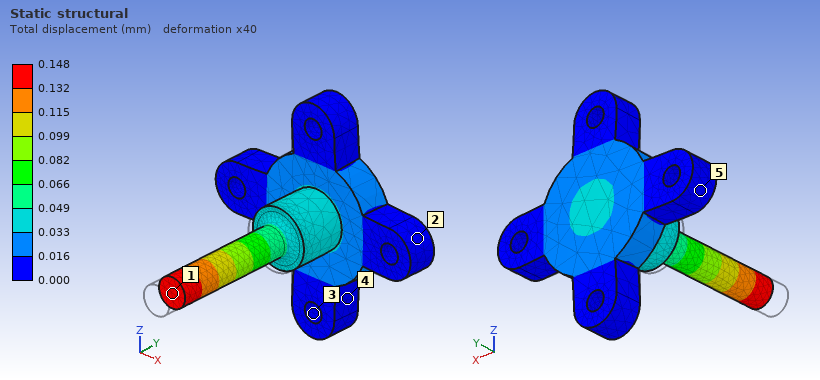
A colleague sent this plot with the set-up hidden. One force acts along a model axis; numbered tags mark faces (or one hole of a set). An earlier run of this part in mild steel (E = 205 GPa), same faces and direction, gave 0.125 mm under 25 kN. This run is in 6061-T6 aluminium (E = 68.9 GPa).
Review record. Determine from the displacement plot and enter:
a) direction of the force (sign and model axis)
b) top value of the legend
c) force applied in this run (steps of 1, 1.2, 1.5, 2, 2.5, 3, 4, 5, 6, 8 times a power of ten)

+Y
0.148 mm
10 kN
